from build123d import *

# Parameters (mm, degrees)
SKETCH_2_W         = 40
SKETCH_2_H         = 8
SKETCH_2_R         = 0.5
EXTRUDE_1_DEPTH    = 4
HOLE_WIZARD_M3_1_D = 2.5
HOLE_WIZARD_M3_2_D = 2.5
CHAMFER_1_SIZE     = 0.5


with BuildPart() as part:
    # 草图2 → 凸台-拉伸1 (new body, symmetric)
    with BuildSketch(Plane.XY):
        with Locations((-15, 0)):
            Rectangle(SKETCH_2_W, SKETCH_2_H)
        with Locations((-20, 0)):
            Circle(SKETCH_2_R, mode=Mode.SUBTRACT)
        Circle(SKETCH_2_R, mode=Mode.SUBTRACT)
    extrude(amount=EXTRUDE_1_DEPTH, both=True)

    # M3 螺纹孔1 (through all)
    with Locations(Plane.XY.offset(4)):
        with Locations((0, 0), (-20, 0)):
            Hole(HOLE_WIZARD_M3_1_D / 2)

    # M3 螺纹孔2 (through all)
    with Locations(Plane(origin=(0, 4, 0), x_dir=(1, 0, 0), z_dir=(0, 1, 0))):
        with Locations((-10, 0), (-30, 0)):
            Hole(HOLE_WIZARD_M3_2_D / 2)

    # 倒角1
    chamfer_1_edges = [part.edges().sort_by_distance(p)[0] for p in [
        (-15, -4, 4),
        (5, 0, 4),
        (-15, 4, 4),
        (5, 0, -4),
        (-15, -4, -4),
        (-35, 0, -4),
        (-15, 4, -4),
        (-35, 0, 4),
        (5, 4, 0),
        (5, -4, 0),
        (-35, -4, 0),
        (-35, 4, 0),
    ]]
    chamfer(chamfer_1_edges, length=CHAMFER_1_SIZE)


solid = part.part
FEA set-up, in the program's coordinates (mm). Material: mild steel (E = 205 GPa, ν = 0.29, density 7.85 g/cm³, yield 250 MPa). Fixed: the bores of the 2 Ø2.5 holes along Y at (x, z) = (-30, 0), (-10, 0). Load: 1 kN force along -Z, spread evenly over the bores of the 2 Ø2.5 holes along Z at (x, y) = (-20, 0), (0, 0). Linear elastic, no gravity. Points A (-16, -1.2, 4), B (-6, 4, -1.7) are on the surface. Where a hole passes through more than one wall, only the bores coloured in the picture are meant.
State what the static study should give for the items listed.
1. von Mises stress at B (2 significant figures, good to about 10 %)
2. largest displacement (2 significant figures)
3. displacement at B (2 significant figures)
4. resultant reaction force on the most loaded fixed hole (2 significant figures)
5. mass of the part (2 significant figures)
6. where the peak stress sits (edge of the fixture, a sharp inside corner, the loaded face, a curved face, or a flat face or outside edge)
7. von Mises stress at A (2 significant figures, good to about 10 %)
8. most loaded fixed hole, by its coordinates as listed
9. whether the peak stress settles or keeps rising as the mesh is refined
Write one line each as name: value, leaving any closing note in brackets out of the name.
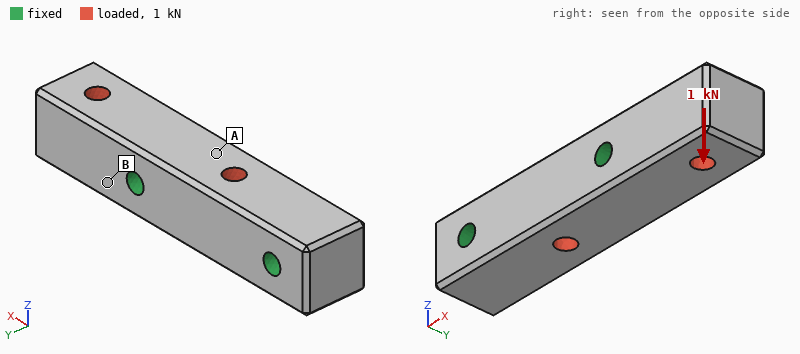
von Mises stress at B: 23 MPa
largest displacement: 7.6 µm
displacement at B: 1.4 µm
resultant reaction force on the most loaded fixed hole: 860 N
mass of the part: 19 g
where the peak stress sits: edge of the fixture
von Mises stress at A: 8.6 MPa
most loaded fixed hole, by its coordinates as listed: (-10, 0)
whether the peak stress settles or keeps rising as the mesh is refined: keeps rising
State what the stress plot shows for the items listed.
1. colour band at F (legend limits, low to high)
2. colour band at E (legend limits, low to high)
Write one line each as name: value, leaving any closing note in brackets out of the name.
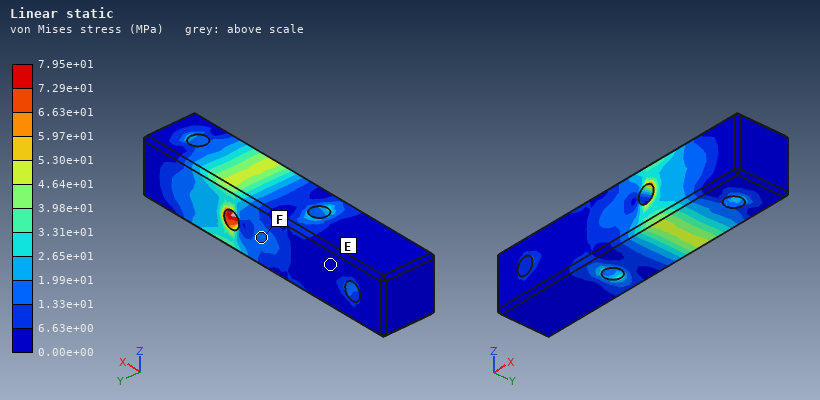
colour band at F: 1.33e+01 to 1.99e+01 MPa
colour band at E: 0.00e+00 to 6.63e+00 MPa
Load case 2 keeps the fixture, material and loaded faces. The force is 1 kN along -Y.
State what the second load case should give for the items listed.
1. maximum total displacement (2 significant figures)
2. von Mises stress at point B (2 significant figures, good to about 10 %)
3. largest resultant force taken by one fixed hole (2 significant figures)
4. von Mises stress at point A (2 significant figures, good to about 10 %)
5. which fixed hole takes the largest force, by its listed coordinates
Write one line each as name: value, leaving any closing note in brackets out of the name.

maximum total displacement: 5.6 µm
von Mises stress at point B: 37 MPa
largest resultant force taken by one fixed hole: 780 N
von Mises stress at point A: 11 MPa
which fixed hole takes the largest force, by its listed coordinates: (-10, 0)
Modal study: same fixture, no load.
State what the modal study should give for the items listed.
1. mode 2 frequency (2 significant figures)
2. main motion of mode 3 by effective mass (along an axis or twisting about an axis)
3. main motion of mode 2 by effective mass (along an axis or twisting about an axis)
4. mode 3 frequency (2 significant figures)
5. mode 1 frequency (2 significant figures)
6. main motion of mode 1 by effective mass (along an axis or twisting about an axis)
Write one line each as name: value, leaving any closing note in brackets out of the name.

mode 2 frequency: 25 kHz
main motion of mode 3 by effective mass: twisting about X
main motion of mode 2 by effective mass: along Y
mode 3 frequency: 49 kHz
mode 1 frequency: 21 kHz
main motion of mode 1 by effective mass: along Z
